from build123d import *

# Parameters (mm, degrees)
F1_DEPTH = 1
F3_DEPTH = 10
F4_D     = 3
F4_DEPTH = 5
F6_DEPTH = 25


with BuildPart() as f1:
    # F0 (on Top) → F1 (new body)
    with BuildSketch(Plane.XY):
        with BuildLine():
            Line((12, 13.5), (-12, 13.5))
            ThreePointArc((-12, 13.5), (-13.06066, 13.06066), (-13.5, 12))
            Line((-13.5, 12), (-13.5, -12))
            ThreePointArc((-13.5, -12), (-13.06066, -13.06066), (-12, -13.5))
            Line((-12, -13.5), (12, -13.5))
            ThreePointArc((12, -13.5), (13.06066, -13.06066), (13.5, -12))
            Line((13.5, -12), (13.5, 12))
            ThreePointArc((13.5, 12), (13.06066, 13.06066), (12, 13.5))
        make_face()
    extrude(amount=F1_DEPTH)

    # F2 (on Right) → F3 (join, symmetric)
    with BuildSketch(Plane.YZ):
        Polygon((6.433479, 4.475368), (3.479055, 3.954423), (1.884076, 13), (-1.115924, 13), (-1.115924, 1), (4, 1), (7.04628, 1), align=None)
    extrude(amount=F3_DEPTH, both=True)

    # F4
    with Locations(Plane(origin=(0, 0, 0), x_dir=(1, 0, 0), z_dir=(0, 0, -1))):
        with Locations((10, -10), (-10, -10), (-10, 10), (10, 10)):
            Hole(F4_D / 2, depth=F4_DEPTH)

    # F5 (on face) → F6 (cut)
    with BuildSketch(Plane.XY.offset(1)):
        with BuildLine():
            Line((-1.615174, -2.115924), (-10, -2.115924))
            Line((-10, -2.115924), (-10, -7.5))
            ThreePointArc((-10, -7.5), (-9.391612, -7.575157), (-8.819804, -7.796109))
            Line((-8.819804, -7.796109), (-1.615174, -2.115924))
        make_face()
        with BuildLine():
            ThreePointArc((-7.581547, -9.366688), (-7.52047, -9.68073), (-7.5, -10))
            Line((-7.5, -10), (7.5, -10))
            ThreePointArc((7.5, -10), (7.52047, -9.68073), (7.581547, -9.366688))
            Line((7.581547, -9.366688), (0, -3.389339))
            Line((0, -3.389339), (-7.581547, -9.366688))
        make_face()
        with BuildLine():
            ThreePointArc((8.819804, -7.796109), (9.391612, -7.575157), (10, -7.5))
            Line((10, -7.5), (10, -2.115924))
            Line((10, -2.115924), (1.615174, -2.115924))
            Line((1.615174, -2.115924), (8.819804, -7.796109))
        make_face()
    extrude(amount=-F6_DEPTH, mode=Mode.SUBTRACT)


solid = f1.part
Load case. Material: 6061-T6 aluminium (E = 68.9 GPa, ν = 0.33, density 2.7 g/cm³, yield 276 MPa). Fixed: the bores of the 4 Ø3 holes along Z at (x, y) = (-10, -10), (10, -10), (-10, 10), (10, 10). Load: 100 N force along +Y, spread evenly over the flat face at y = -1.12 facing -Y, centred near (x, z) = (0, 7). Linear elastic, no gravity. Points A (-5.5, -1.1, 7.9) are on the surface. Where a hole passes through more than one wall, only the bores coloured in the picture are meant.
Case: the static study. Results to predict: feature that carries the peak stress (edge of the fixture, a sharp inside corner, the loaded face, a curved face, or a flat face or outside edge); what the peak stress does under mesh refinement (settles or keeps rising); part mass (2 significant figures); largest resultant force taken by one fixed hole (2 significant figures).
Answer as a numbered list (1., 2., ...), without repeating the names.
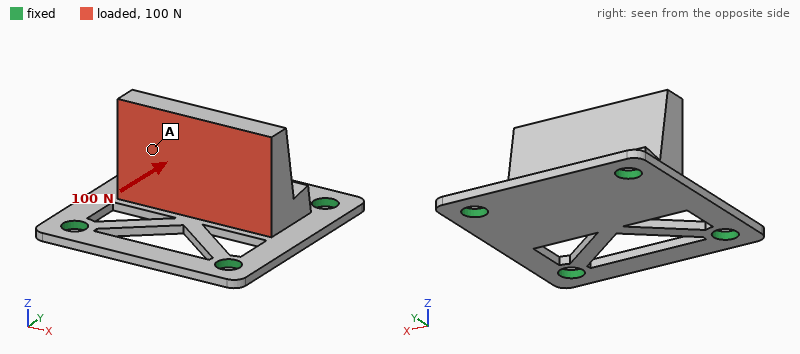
1. a sharp inside corner
2. keeps rising
3. 4.8 g
4. 50 N
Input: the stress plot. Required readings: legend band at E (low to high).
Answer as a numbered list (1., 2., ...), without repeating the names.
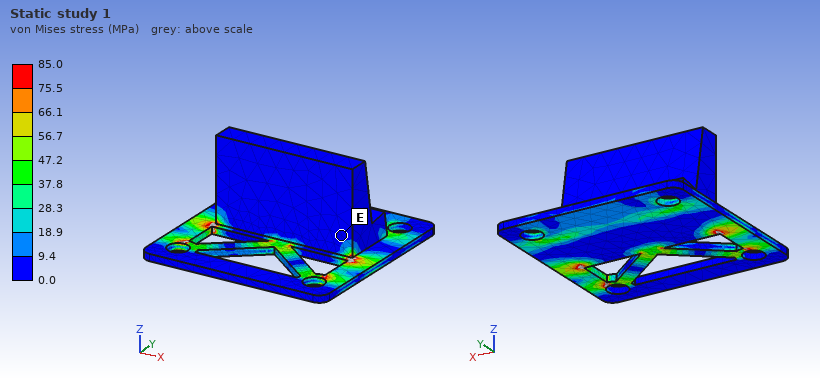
1. 0.0 to 9.4 MPa
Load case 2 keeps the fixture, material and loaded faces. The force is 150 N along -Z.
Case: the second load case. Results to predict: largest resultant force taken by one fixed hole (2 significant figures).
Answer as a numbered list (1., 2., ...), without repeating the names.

1. 39 N
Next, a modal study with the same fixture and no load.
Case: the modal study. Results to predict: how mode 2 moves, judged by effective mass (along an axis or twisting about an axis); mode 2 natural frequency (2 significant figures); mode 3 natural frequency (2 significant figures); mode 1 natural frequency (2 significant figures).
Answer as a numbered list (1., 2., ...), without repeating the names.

1. along X
2. 12 kHz
3. 16 kHz
4. 4100 Hz
